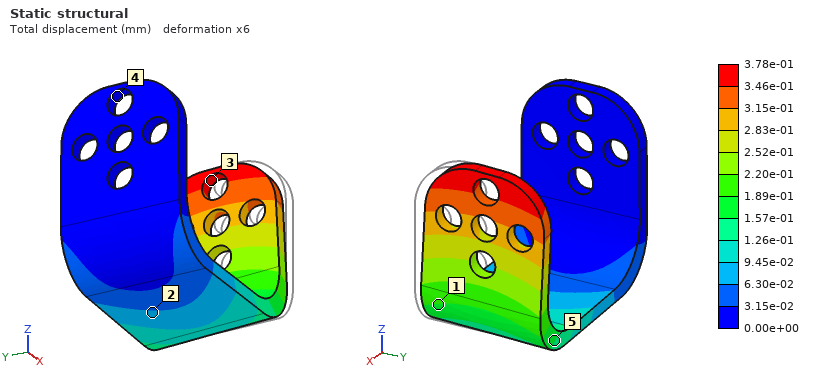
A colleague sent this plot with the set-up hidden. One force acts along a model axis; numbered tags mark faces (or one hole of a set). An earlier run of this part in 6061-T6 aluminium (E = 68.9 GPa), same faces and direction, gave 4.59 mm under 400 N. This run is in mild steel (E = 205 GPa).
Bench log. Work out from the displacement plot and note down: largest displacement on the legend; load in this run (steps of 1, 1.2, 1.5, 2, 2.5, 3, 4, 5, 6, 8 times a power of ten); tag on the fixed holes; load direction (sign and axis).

3.78e-01 mm
100 N
4
+Y
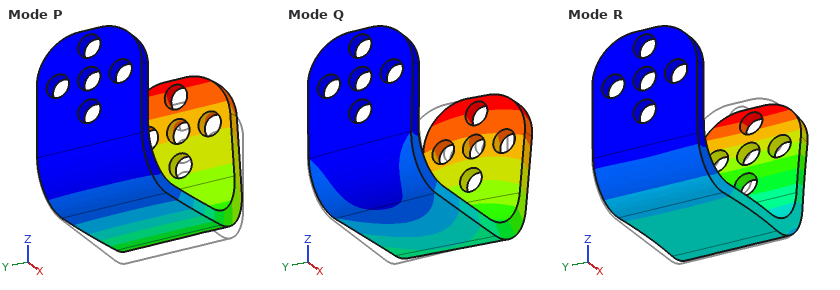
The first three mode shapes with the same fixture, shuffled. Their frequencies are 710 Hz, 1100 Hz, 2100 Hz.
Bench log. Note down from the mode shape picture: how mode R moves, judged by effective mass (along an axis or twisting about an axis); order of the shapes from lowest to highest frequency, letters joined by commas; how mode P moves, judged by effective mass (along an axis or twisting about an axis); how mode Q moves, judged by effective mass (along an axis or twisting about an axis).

along X
P, Q, R
along Z
along Y
